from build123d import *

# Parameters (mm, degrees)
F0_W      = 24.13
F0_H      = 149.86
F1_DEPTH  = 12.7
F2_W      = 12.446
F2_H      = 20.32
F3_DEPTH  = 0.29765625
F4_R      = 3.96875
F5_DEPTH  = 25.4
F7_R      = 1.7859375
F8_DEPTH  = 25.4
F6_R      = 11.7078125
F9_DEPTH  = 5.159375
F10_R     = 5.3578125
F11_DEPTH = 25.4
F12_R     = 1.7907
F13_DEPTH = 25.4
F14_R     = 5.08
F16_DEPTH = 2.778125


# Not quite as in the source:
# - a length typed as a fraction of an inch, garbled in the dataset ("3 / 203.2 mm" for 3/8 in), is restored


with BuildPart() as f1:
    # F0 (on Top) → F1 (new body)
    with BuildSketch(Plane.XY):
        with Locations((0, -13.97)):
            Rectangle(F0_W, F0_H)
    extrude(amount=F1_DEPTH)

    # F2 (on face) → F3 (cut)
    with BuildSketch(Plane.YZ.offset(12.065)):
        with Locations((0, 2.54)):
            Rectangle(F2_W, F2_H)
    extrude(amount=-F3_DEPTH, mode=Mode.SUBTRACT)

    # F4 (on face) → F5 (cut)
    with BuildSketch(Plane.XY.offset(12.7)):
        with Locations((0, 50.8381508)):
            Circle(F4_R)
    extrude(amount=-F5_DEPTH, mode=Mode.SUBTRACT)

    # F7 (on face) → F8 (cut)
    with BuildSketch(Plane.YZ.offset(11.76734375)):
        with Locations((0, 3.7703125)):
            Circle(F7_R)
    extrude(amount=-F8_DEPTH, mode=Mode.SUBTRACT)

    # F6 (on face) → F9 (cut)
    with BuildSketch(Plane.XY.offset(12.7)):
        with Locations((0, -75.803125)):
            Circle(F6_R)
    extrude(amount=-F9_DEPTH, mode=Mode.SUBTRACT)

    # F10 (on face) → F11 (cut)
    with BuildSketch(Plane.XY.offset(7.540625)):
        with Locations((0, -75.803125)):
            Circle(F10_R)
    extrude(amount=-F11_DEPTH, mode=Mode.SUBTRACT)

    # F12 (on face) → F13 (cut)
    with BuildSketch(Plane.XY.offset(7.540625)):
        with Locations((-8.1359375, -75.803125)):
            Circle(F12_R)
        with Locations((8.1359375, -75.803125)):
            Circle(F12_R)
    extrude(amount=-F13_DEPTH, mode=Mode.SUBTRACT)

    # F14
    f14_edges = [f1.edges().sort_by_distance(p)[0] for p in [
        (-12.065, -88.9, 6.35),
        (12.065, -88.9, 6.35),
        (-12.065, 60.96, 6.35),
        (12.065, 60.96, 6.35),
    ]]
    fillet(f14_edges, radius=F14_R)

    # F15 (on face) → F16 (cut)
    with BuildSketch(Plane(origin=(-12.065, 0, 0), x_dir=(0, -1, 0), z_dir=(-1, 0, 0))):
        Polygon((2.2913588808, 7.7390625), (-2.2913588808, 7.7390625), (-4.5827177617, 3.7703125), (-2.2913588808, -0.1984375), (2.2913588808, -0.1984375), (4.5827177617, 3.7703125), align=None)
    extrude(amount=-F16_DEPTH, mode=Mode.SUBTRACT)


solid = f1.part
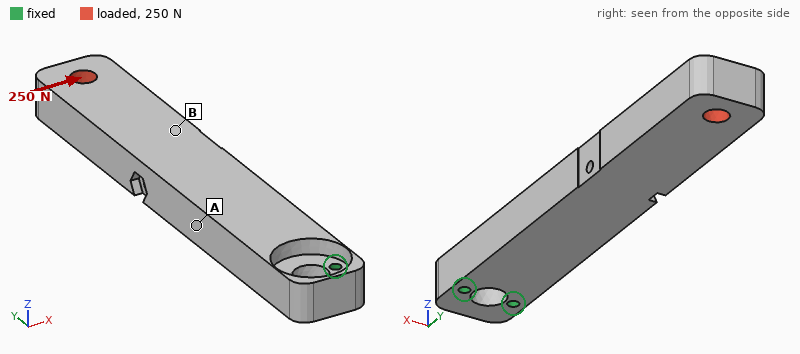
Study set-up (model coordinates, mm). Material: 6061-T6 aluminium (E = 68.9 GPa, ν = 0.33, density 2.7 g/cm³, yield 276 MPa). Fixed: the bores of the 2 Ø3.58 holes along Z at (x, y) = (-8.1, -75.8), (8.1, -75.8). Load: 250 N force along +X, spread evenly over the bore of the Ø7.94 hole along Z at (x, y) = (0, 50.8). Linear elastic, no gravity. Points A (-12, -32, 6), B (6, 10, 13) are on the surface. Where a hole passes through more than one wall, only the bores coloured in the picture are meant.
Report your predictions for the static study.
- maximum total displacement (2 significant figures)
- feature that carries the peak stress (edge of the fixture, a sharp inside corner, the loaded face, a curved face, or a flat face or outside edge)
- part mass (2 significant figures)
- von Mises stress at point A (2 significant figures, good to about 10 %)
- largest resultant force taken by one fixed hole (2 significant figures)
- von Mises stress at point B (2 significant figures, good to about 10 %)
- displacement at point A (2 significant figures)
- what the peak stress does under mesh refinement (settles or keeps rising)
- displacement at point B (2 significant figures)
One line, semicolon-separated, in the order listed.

0.23 mm; edge of the fixture; 110 g; 17 MPa; 1.8 kN; 5.8 MPa; 0.039 mm; keeps rising; 0.11 mm
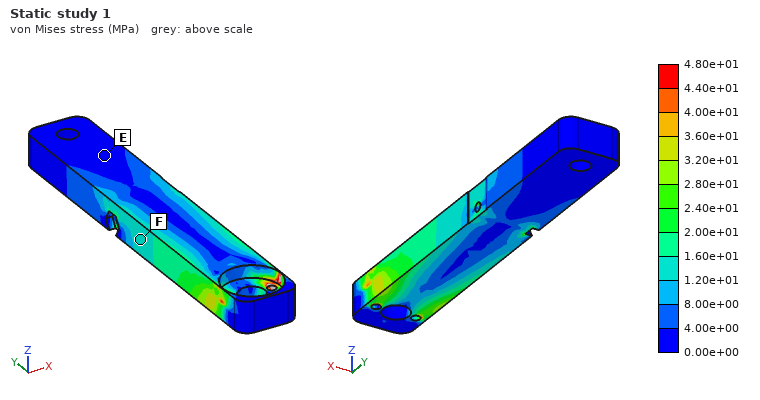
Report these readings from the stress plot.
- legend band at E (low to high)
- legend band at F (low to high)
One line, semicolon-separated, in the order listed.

0.00e+00 to 4.00e+00 MPa; 1.20e+01 to 1.60e+01 MPa
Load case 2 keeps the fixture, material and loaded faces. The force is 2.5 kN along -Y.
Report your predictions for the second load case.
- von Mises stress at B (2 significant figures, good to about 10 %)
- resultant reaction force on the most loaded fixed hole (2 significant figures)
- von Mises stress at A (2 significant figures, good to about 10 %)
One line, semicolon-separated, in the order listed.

8.0 MPa; 1.3 kN; 8.1 MPa
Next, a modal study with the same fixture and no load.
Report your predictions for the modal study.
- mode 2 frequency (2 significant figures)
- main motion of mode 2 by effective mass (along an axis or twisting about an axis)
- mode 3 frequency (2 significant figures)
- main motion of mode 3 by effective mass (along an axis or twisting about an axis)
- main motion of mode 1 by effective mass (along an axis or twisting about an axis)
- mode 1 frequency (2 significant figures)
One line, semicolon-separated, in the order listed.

970 Hz; along X; 2800 Hz; along Z; along Z; 400 Hz
